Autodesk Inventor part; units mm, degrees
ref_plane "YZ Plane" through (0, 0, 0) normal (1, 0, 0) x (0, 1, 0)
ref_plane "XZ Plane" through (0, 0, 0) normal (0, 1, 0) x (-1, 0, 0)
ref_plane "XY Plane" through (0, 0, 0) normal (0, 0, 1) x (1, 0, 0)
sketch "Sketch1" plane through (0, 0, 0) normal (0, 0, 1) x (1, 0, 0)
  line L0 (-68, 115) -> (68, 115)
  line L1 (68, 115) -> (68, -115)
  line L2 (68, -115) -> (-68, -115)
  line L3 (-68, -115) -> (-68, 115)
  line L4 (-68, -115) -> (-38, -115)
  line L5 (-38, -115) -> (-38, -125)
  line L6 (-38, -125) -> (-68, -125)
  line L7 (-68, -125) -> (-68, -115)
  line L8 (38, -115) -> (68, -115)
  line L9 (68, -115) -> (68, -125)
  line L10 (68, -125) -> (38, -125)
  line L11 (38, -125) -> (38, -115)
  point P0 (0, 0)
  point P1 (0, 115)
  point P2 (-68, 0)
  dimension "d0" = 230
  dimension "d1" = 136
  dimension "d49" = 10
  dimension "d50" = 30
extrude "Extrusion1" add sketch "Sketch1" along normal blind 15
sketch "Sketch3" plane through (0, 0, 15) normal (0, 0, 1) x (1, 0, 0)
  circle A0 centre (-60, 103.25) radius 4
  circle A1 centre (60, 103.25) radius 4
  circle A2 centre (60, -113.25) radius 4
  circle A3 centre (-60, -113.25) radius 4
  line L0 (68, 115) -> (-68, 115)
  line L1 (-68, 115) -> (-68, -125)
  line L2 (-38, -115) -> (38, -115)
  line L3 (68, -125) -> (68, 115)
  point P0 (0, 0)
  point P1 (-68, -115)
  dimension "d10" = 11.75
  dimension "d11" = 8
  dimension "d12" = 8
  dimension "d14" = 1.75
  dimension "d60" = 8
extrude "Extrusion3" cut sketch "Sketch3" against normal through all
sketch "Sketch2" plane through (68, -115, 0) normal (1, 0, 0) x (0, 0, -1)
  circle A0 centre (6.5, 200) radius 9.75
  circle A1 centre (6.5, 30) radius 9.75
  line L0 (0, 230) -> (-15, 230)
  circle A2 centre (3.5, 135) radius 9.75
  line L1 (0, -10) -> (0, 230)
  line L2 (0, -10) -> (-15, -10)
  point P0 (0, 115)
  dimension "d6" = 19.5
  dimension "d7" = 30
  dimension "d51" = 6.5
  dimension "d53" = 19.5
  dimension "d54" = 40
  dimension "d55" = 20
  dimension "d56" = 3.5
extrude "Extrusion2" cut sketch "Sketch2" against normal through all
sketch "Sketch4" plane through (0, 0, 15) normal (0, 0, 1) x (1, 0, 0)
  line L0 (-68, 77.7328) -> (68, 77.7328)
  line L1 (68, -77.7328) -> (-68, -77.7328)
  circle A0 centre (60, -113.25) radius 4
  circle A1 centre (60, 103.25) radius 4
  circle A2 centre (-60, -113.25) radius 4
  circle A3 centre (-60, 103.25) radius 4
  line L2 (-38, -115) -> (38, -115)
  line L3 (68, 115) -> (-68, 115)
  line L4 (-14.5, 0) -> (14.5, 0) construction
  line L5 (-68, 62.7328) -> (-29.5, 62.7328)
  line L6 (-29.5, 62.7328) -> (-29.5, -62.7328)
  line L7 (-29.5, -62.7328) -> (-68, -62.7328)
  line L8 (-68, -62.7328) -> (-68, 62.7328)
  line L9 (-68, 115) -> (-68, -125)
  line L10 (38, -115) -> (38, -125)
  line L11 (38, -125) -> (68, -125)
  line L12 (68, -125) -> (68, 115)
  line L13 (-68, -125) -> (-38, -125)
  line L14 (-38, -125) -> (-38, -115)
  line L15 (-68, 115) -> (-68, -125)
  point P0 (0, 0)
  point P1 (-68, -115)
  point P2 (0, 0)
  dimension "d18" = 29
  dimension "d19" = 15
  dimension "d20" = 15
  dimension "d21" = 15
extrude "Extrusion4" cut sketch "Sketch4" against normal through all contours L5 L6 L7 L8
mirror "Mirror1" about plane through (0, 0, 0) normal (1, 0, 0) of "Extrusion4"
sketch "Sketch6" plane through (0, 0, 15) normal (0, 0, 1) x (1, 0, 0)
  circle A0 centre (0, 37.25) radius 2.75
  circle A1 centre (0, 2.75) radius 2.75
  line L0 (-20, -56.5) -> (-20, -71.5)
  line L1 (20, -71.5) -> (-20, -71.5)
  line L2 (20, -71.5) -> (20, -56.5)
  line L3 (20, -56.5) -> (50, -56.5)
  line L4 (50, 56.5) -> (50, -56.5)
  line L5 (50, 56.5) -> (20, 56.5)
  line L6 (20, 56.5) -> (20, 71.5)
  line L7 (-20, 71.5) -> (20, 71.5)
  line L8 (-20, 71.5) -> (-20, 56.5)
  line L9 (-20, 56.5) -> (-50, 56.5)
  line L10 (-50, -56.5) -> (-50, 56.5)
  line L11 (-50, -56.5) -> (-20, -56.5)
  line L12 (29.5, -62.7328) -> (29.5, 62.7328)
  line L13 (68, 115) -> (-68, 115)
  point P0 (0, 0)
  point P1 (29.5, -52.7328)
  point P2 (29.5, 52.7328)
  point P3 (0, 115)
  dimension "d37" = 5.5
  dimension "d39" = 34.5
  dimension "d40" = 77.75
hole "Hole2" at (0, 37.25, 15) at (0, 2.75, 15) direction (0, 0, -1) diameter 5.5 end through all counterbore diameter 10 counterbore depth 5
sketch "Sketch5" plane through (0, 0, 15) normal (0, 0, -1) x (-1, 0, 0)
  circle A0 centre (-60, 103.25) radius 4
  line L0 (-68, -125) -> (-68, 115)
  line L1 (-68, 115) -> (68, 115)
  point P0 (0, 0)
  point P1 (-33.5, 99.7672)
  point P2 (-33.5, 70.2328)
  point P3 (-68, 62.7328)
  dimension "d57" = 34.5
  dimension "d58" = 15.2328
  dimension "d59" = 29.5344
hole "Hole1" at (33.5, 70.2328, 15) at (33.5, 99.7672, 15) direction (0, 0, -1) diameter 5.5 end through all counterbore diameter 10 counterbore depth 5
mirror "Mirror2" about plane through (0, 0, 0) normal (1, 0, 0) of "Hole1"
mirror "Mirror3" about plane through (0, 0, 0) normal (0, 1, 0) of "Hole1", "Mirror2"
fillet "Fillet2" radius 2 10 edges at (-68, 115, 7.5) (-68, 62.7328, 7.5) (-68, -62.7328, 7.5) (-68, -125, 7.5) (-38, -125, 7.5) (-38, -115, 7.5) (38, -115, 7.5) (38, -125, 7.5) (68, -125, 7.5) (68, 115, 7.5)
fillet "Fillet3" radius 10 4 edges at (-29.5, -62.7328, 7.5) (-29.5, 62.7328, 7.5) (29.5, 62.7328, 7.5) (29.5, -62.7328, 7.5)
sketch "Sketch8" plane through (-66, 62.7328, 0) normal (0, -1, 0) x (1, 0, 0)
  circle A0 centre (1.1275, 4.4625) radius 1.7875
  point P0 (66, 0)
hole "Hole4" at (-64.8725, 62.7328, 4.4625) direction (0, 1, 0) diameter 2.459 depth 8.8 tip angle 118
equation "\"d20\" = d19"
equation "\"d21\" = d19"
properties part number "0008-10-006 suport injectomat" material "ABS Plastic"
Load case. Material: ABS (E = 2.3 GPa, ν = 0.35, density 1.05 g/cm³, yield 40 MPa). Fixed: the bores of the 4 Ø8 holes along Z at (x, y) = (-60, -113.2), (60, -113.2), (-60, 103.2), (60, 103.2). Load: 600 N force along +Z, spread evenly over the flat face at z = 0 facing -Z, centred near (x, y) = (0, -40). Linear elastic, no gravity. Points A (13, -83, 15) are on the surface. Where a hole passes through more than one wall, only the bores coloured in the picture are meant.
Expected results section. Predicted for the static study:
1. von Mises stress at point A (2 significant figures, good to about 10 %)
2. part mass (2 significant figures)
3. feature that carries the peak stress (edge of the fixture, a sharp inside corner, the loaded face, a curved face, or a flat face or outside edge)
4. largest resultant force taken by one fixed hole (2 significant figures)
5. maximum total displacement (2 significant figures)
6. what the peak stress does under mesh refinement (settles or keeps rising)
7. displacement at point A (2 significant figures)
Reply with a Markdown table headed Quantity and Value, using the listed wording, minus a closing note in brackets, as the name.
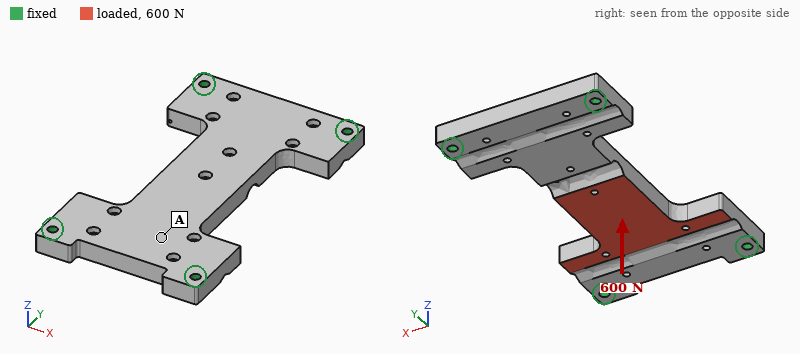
| Quantity | Value |
|---|---|
| von Mises stress at point A | 1.6 MPa |
| part mass | 330 g |
| feature that carries the peak stress | edge of the fixture |
| largest resultant force taken by one fixed hole | 220 N |
| maximum total displacement | 0.84 mm |
| what the peak stress does under mesh refinement | keeps rising |
| displacement at point A | 0.32 mm |
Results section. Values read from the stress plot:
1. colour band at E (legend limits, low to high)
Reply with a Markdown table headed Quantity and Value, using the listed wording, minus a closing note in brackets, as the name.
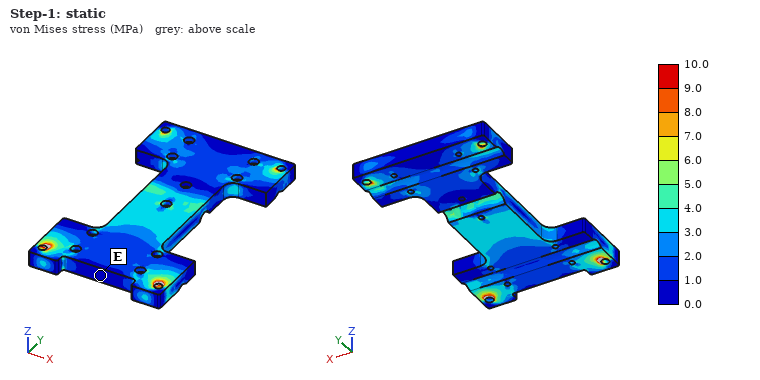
| Quantity | Value |
|---|---|
| colour band at E | 0.0 to 1.0 MPa |
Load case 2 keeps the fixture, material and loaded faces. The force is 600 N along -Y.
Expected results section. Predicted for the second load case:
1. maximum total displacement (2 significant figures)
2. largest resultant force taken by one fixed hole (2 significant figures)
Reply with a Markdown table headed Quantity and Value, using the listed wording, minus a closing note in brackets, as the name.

| Quantity | Value |
|---|---|
| maximum total displacement | 99 µm |
| largest resultant force taken by one fixed hole | 240 N |
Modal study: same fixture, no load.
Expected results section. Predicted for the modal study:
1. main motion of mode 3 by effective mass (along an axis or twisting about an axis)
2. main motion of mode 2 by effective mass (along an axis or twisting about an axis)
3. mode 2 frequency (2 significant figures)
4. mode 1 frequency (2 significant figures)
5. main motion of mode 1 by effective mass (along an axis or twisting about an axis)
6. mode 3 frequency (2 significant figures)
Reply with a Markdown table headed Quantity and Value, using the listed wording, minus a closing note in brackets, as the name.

| Quantity | Value |
|---|---|
| main motion of mode 3 by effective mass | twisting about Y |
| main motion of mode 2 by effective mass | twisting about X |
| mode 2 frequency | 900 Hz |
| mode 1 frequency | 380 Hz |
| main motion of mode 1 by effective mass | along Z |
| mode 3 frequency | 1100 Hz |
